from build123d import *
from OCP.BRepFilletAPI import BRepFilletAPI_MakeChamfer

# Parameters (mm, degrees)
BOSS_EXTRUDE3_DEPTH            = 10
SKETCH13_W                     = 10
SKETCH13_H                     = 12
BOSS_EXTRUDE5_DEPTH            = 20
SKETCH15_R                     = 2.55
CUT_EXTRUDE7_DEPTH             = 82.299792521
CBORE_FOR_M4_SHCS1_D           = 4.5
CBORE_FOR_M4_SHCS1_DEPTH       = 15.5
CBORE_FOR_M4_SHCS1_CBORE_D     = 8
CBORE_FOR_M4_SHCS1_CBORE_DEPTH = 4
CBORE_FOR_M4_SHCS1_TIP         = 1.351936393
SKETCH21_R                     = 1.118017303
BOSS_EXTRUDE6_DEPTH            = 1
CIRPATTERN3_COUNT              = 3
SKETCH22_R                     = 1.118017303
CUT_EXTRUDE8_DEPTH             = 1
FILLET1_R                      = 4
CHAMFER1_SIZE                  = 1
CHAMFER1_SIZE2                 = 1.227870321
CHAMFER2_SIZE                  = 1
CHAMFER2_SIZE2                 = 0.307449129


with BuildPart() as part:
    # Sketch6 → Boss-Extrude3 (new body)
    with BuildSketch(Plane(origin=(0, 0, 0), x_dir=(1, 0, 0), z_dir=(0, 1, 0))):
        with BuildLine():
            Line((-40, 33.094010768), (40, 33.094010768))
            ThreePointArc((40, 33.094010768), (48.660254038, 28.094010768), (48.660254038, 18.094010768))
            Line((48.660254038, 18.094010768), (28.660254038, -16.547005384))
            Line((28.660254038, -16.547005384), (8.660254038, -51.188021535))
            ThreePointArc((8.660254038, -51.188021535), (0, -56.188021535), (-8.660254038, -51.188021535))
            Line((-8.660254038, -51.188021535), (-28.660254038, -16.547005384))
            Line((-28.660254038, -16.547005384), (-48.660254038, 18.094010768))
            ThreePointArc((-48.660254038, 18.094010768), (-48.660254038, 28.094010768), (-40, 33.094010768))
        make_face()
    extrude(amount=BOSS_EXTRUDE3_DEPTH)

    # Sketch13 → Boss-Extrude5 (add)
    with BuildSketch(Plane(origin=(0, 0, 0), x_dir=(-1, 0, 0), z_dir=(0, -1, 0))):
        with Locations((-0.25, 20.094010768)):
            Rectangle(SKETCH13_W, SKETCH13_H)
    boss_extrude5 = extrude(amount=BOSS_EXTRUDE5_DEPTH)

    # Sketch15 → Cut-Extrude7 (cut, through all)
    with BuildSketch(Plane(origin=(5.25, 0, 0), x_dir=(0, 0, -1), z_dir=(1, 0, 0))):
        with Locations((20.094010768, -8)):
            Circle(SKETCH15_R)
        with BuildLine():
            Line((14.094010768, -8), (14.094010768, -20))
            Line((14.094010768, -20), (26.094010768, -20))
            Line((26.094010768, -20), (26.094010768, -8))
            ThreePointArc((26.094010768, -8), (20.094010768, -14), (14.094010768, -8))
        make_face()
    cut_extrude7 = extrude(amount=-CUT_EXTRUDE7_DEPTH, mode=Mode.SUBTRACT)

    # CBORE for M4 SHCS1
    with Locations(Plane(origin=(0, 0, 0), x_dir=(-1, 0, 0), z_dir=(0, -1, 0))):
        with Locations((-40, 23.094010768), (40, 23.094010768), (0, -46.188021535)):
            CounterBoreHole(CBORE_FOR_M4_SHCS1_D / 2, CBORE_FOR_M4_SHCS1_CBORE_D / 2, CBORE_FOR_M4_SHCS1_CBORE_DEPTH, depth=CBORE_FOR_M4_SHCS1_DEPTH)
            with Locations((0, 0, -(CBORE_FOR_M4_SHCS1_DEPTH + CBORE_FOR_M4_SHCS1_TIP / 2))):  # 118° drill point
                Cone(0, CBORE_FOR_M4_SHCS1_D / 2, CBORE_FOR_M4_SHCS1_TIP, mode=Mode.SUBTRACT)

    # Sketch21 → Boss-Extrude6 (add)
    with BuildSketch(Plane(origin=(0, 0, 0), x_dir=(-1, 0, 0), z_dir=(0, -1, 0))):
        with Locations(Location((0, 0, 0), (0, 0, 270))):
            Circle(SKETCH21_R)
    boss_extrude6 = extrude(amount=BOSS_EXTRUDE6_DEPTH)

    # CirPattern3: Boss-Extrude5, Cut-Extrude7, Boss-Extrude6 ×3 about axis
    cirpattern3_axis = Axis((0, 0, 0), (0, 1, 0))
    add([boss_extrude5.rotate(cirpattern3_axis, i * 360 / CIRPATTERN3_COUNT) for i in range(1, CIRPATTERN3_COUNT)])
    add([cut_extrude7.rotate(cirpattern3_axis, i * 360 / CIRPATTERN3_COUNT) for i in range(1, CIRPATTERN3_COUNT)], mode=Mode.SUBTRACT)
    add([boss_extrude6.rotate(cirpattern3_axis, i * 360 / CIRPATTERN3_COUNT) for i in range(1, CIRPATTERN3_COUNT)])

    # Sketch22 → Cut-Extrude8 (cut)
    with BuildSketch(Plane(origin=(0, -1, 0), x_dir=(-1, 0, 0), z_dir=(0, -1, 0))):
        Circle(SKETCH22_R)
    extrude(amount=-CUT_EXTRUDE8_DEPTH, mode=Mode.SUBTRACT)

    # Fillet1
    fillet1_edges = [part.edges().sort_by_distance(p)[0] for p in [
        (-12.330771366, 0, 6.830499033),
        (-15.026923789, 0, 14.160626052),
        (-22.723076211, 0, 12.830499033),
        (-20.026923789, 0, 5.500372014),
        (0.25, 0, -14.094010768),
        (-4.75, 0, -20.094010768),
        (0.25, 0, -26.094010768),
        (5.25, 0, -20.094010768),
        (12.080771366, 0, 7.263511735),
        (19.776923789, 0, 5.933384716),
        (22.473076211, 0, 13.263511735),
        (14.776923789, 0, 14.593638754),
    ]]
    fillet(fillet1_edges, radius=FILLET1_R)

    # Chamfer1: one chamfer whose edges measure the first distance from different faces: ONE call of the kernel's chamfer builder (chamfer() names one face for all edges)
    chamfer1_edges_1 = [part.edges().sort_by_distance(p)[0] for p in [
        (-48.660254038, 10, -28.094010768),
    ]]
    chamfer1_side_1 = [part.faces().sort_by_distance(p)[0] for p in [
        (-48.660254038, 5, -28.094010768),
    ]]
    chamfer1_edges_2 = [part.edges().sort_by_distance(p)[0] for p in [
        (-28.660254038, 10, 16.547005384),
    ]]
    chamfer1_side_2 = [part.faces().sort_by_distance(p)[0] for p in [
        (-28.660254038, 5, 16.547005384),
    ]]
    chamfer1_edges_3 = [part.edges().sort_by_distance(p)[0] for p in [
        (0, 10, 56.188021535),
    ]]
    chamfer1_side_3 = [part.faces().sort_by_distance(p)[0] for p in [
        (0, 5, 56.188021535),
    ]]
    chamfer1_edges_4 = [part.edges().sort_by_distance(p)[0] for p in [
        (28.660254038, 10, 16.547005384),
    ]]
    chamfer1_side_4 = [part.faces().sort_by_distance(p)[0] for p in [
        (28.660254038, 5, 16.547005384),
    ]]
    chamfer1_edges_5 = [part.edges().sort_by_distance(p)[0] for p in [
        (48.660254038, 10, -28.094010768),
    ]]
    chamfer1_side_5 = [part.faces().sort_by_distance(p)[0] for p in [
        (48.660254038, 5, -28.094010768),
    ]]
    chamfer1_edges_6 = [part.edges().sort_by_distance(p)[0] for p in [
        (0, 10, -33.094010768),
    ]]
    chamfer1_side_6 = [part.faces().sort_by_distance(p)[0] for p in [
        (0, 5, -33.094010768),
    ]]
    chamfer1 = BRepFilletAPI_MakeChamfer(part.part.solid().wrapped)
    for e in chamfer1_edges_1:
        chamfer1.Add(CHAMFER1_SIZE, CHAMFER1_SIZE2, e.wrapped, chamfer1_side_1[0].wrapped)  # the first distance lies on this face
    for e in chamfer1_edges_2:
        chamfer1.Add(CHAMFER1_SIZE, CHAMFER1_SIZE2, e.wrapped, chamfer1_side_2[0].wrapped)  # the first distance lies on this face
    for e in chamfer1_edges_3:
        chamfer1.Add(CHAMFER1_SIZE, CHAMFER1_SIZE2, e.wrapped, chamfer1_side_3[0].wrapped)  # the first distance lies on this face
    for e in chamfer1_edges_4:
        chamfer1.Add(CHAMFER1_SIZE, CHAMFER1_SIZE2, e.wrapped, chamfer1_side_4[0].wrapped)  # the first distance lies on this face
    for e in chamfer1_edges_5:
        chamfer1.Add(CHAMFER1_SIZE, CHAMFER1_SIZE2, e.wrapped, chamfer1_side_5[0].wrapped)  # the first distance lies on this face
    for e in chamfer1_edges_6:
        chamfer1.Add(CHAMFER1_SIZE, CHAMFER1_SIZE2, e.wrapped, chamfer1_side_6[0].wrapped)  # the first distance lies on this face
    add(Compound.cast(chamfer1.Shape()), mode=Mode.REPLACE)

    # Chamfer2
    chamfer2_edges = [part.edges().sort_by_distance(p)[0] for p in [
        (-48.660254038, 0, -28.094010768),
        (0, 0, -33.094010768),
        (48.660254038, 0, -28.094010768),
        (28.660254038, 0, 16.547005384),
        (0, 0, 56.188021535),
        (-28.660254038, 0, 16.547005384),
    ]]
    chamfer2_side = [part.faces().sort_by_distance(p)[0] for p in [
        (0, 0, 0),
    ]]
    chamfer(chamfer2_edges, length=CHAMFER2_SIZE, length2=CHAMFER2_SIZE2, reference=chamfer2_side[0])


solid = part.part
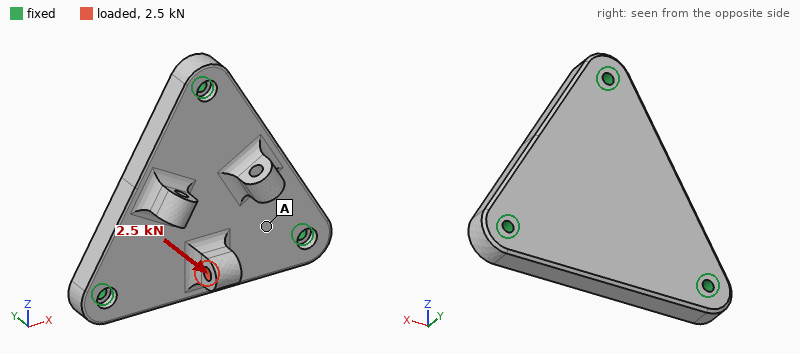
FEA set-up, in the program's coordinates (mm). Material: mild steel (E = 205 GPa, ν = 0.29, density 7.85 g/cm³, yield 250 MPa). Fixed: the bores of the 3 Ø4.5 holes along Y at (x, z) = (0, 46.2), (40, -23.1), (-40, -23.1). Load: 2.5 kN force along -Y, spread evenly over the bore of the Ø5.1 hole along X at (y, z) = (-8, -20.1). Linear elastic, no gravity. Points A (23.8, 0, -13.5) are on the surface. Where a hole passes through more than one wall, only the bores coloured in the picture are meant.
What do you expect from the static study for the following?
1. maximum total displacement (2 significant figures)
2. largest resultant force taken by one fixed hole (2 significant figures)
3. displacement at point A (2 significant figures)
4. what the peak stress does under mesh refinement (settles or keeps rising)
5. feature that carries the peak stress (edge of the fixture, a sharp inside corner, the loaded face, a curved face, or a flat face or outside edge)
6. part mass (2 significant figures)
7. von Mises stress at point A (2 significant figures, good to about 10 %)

21 µm
1.6 kN
7.9 µm
keeps rising
edge of the fixture
460 g
18 MPa
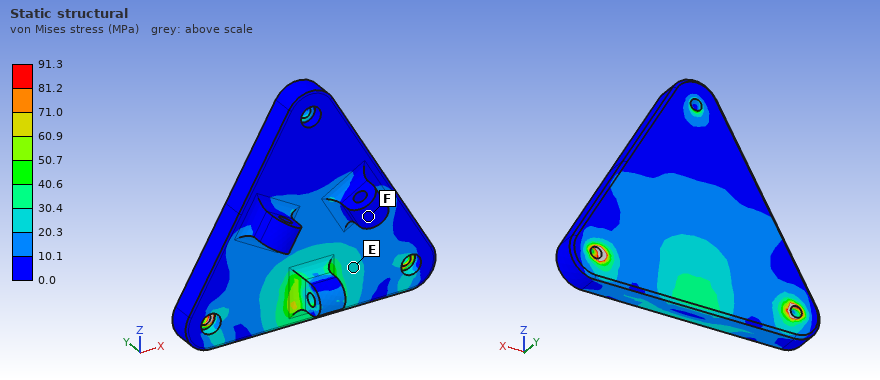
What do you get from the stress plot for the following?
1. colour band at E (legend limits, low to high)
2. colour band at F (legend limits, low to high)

20.3 to 30.4 MPa
0.0 to 10.1 MPa
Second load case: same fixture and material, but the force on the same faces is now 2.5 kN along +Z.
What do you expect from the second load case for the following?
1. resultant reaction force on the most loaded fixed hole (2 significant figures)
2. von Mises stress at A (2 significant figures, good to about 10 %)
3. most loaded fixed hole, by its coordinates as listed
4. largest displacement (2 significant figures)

1.6 kN
15 MPa
(0, 46.2)
20 µm
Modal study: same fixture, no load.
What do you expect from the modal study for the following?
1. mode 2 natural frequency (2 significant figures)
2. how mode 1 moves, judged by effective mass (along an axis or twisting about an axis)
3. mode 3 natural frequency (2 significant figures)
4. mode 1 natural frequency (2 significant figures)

7300 Hz
along Y
7300 Hz
4900 Hz
